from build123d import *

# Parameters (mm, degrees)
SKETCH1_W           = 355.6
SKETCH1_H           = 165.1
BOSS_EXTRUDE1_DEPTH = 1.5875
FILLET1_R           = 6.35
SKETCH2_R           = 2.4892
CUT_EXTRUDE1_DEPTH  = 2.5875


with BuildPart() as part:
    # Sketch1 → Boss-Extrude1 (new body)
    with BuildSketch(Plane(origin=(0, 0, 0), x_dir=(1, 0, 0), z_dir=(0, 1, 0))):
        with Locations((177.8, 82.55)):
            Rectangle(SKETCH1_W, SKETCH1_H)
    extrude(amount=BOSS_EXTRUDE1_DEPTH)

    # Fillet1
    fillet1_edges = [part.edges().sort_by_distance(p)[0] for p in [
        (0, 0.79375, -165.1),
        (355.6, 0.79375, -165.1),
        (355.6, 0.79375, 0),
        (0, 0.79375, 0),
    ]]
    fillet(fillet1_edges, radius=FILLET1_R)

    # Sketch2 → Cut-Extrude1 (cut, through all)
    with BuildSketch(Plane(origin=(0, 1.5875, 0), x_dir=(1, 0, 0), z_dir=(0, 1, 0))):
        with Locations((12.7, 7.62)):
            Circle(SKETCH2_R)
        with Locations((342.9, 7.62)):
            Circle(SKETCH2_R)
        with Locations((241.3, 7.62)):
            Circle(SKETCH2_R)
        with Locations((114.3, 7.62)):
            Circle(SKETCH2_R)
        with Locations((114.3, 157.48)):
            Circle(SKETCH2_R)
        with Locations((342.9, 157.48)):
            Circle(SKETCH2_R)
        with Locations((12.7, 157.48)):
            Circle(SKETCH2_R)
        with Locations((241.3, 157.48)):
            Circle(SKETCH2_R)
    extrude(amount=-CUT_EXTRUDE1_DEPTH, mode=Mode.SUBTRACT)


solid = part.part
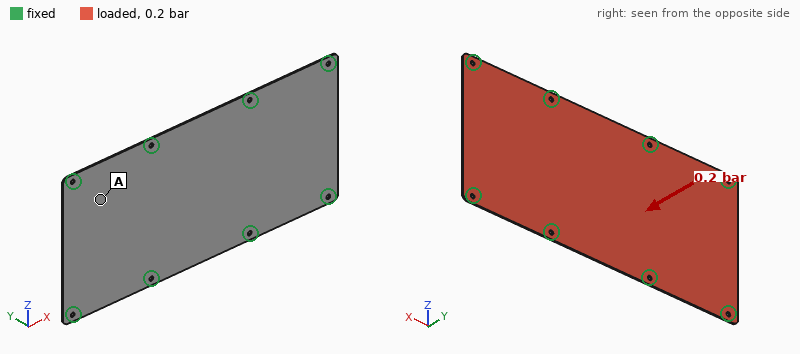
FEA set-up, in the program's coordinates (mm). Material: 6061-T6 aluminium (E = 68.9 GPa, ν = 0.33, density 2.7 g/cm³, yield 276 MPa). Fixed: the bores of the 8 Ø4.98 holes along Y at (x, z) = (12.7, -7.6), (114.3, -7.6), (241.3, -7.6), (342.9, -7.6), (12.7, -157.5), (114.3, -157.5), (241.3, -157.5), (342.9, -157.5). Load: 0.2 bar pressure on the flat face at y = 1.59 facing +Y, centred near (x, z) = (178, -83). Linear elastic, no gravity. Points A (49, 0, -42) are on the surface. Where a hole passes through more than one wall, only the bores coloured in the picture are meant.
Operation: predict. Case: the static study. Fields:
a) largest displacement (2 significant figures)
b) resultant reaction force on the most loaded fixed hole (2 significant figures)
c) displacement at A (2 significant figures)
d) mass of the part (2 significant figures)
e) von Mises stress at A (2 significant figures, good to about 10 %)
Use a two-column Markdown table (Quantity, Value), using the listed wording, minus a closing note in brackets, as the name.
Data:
| Quantity | Value |
|---|---|
| largest displacement | 2.3 mm |
| resultant reaction force on the most loaded fixed hole | 190 N |
| displacement at A | 1.1 mm |
| mass of the part | 250 g |
| von Mises stress at A | 23 MPa |
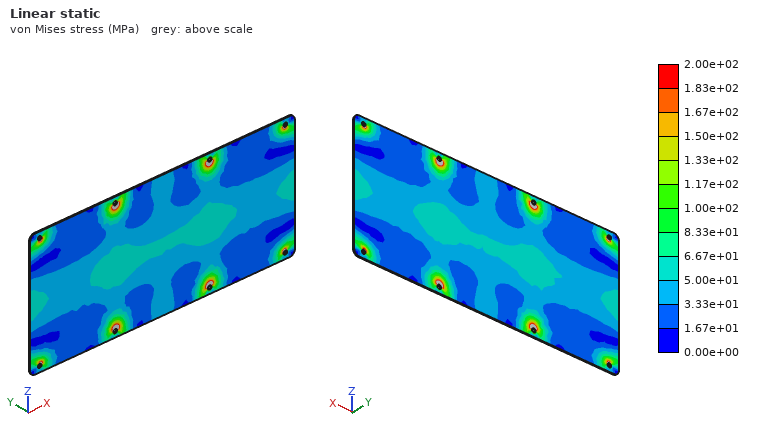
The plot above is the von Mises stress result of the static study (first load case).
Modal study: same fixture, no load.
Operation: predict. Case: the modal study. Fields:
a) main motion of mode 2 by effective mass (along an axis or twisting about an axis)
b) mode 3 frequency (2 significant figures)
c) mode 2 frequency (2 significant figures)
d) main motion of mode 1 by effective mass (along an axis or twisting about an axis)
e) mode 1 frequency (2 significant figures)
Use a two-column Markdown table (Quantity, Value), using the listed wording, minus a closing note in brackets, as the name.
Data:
| Quantity | Value |
|---|---|
| main motion of mode 2 by effective mass | twisting about Z |
| mode 3 frequency | 350 Hz |
| mode 2 frequency | 320 Hz |
| main motion of mode 1 by effective mass | along Y |
| mode 1 frequency | 280 Hz |
